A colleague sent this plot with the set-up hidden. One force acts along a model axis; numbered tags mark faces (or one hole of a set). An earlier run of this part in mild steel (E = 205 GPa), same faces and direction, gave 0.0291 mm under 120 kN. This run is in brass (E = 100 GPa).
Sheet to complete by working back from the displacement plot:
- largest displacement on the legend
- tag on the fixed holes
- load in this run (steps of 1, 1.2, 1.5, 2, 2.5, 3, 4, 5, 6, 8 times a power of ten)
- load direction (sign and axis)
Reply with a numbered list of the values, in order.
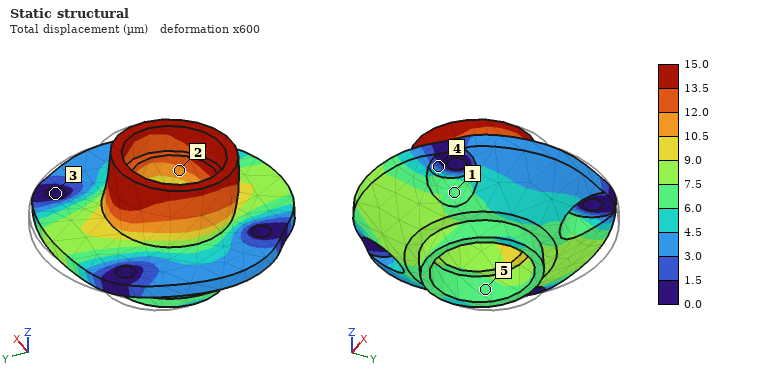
1. 15.0 µm
2. 3
3. 30 kN
4. -Y
